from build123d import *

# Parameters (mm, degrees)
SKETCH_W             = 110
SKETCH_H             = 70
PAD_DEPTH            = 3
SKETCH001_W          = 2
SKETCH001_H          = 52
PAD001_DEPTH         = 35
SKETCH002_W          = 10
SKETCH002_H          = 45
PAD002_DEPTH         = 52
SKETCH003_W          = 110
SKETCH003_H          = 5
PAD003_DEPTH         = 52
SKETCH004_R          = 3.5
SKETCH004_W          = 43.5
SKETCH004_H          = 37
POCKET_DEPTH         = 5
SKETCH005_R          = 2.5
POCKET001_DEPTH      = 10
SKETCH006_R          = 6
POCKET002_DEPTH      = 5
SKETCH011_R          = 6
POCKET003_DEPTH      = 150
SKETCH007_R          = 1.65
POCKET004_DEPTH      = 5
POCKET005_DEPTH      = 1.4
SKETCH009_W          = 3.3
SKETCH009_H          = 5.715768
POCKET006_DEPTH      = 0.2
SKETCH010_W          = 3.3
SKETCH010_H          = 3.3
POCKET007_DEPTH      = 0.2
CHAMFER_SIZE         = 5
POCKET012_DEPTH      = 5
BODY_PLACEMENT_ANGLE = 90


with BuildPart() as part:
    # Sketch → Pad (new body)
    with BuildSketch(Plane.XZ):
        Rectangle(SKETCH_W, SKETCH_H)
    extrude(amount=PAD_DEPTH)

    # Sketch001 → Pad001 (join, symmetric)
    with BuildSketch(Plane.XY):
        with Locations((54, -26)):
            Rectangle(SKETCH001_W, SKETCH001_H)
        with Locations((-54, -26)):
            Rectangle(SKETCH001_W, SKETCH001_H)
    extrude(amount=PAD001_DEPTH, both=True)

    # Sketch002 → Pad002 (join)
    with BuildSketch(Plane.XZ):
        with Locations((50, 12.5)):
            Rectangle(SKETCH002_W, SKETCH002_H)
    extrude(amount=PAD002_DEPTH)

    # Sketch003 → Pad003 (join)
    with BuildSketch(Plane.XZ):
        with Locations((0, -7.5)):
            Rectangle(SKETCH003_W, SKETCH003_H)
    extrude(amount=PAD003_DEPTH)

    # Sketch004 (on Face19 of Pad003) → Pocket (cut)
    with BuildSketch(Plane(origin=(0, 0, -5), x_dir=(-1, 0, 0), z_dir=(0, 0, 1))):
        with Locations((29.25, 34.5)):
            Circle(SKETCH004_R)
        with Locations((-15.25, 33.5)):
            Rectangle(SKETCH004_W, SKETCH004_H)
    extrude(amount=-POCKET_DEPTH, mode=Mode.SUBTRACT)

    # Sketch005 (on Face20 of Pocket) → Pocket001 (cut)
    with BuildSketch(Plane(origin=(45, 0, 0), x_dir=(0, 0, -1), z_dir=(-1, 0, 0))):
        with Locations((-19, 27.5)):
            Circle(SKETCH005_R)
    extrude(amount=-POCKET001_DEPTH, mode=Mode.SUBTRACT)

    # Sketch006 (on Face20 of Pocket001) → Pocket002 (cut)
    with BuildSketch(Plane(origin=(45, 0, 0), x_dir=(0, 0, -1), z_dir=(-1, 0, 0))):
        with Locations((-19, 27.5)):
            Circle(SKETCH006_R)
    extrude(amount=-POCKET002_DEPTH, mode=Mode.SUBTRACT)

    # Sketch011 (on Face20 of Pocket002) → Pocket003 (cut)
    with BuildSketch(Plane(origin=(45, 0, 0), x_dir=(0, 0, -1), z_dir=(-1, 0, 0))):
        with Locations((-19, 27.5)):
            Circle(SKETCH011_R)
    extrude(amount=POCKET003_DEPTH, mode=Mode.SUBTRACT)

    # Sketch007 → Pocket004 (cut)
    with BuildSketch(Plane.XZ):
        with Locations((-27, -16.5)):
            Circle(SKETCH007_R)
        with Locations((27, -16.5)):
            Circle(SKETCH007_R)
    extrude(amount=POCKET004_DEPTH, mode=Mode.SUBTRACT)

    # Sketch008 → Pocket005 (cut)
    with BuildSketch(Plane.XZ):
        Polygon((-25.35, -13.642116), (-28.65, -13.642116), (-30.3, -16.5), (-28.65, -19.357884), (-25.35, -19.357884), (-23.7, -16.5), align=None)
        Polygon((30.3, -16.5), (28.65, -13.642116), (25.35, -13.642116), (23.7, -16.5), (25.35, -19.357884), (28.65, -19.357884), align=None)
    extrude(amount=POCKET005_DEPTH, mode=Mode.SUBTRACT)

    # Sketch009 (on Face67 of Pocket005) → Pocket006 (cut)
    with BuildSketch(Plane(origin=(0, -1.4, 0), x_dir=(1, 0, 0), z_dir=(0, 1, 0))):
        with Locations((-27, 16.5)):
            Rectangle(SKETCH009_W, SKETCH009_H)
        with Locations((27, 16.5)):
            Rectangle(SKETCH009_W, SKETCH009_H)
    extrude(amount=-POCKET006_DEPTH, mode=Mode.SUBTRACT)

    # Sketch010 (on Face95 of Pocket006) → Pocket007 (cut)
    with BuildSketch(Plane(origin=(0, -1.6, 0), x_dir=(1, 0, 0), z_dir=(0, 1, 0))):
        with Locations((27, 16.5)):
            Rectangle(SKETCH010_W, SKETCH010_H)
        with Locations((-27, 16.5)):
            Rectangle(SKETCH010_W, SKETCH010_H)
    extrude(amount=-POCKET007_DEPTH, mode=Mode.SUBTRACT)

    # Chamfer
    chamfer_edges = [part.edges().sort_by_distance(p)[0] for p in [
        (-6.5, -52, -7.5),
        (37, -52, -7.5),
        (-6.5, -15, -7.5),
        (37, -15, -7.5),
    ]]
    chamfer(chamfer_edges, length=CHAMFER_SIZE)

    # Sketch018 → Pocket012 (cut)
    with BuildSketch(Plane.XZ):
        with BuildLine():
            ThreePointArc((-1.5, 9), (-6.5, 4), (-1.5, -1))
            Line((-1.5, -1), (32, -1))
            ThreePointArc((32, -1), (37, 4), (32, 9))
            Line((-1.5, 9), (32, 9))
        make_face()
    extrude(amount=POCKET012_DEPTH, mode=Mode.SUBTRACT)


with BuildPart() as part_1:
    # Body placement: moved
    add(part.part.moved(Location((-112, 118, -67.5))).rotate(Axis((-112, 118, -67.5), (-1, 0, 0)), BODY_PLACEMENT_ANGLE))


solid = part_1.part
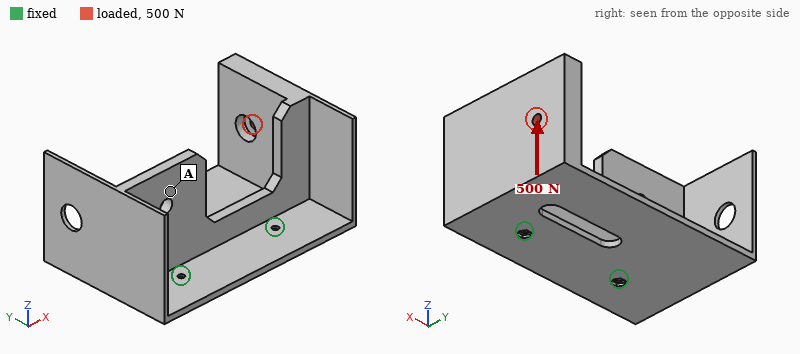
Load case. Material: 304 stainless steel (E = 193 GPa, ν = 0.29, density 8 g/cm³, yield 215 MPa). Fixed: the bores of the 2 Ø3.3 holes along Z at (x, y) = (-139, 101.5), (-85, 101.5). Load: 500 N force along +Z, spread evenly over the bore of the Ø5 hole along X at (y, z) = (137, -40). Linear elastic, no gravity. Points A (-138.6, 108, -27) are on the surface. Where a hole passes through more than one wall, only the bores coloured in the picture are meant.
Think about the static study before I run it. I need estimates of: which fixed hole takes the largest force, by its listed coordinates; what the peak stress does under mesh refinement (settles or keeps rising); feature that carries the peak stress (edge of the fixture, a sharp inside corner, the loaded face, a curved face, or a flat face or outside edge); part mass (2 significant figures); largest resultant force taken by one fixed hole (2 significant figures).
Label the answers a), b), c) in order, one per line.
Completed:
a) (-85, 101.5)
b) keeps rising
c) edge of the fixture
d) 540 g
e) 780 N
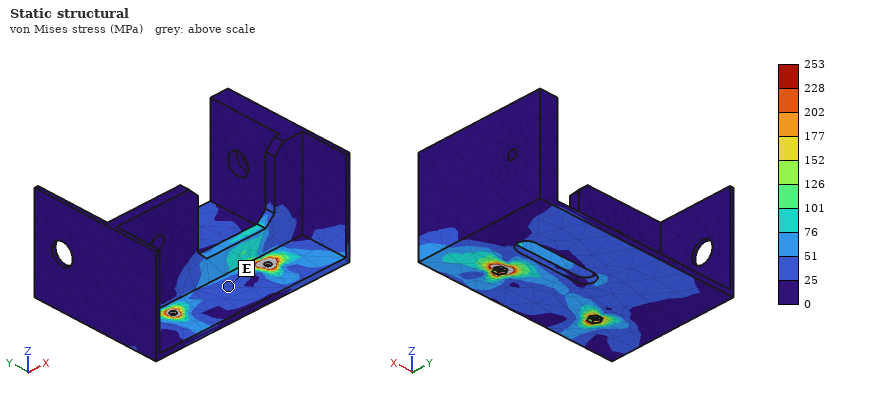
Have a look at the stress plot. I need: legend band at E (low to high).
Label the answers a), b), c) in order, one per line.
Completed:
a) 25 to 51 MPa
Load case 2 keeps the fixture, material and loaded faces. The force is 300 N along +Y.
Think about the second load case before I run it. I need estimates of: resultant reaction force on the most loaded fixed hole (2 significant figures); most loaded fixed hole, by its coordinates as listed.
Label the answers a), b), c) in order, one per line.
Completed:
a) 440 N
b) (-85, 101.5)
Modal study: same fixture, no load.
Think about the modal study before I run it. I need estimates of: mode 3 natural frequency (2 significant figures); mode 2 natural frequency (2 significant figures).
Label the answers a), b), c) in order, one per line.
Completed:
a) 1100 Hz
b) 530 Hz
